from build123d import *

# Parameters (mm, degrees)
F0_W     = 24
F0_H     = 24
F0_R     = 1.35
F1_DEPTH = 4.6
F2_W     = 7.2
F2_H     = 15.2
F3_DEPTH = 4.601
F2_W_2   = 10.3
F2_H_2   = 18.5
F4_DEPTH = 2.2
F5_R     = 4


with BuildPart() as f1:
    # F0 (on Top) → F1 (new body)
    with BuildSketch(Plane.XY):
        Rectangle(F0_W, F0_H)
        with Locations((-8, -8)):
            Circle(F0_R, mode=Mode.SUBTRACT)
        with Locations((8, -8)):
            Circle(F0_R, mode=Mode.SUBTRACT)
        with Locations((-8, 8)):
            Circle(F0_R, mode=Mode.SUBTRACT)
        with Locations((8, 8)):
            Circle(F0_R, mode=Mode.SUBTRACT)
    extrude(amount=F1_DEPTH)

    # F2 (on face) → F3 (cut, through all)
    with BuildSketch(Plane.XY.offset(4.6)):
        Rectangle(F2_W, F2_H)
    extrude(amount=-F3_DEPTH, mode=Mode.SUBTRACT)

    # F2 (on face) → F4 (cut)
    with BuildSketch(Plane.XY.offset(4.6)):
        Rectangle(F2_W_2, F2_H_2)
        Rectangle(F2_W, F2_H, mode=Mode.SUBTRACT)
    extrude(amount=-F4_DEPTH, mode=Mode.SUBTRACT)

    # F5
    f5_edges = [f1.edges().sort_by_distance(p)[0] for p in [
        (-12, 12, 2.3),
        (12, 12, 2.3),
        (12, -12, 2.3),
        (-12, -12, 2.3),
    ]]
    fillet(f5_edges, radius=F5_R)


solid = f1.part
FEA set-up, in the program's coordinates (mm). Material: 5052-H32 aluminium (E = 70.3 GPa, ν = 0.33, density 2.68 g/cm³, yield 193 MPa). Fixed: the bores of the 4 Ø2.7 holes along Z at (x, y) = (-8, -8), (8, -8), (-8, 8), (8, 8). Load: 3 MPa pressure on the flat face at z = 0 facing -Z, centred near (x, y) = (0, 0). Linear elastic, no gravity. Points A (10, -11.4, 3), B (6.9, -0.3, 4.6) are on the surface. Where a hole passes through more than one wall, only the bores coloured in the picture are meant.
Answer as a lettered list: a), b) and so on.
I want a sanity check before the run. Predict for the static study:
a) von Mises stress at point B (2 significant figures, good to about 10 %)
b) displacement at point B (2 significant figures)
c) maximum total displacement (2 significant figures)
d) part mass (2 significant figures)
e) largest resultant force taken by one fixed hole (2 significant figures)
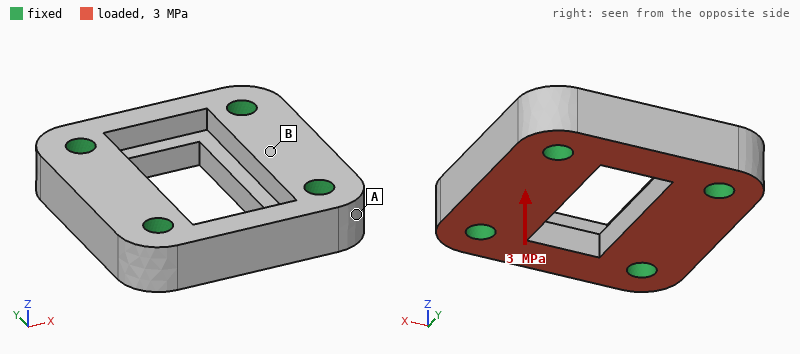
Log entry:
a) 9.7 MPa
b) 1.7 µm
c) 2.5 µm
d) 4.8 g
e) 320 N
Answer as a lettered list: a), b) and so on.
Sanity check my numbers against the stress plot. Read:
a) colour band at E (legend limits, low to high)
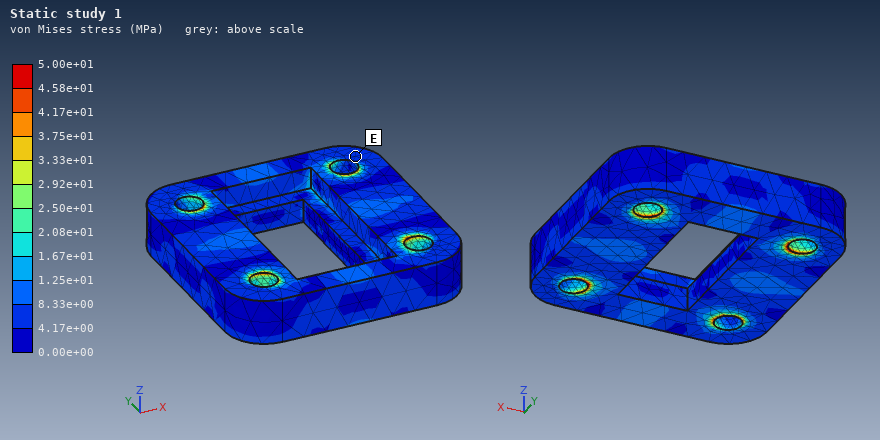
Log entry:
a) 4.17e+00 to 8.33e+00 MPa
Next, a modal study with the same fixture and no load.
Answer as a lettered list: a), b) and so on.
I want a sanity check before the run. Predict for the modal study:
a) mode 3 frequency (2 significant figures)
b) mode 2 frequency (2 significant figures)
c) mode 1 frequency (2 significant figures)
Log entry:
a) 71 kHz
b) 69 kHz
c) 69 kHz
